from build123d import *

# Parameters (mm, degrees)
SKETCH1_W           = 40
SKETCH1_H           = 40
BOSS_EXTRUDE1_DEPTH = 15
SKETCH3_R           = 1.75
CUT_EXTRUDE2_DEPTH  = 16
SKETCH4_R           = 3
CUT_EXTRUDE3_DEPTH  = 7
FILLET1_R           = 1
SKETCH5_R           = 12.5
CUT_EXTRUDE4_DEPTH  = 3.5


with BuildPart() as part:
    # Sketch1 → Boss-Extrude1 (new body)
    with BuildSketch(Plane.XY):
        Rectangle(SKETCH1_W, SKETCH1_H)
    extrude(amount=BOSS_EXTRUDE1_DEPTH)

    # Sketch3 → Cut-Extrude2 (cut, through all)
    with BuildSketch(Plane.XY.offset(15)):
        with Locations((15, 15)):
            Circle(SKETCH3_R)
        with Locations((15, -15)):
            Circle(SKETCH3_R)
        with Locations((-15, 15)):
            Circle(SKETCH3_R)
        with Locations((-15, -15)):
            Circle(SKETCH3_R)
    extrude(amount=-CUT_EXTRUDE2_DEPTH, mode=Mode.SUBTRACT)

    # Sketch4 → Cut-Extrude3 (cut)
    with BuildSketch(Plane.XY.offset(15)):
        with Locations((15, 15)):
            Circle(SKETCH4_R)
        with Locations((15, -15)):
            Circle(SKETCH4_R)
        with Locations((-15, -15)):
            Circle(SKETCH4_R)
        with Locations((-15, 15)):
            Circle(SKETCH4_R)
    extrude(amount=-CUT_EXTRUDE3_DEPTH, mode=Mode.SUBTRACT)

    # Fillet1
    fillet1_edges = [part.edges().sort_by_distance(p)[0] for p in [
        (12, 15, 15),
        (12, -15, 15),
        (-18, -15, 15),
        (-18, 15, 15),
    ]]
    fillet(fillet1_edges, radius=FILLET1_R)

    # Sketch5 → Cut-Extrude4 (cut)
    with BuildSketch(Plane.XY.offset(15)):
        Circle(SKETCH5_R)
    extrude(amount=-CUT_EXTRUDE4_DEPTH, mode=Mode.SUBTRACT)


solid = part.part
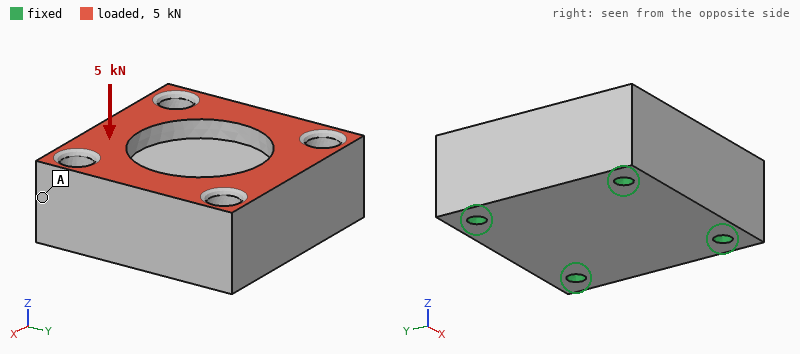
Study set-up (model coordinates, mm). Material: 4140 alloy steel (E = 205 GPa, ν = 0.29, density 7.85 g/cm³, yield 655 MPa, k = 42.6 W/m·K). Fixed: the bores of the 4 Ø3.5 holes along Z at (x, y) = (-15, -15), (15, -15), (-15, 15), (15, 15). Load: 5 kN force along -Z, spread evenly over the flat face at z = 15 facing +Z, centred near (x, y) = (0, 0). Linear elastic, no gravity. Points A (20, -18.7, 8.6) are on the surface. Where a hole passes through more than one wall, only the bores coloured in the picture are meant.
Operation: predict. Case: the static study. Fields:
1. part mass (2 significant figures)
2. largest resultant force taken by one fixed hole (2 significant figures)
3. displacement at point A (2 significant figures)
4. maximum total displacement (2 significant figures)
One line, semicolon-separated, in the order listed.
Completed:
170 g; 1.3 kN; 0.17 µm; 1.1 µm
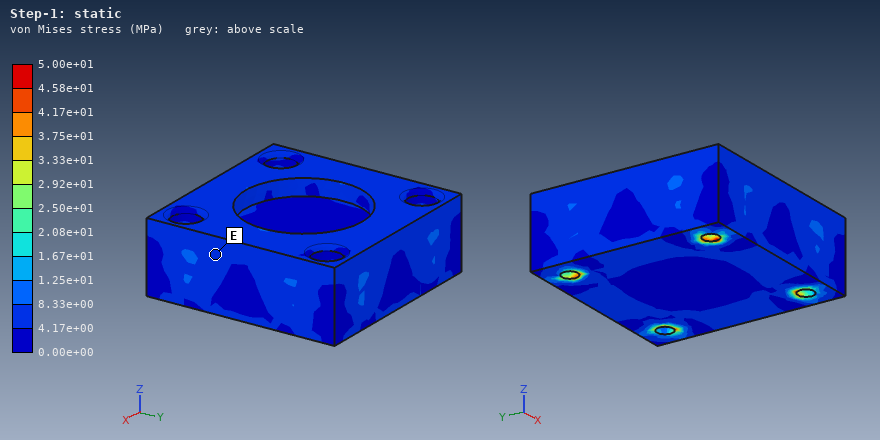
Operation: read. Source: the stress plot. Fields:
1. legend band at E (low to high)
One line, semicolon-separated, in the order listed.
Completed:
4.17e+00 to 8.33e+00 MPa
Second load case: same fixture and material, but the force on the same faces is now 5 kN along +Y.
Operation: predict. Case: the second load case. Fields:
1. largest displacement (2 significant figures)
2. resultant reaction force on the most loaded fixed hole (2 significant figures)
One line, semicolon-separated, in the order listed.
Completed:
2.6 µm; 1.5 kN
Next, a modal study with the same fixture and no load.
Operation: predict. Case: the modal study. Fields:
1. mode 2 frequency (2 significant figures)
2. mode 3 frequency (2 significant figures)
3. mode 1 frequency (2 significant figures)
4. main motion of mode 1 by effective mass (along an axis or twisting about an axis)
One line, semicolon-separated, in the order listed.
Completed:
35 kHz; 35 kHz; 27 kHz; along Z
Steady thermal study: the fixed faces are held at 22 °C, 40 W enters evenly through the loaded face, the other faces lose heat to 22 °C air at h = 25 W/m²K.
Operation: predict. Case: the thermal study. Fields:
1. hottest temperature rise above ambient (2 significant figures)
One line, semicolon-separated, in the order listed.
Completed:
17 K
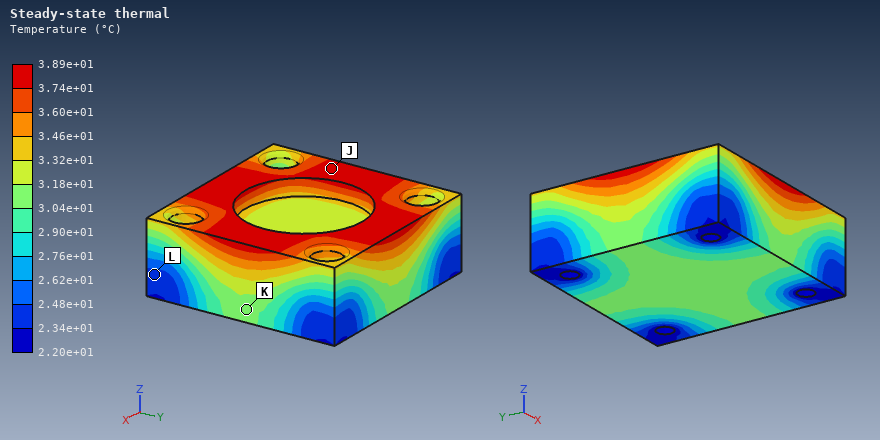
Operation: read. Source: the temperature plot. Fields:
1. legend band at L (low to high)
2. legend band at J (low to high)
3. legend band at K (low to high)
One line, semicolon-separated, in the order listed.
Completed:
2.34e+01 to 2.48e+01 °C; 3.74e+01 to 3.89e+01 °C; 3.04e+01 to 3.18e+01 °C
